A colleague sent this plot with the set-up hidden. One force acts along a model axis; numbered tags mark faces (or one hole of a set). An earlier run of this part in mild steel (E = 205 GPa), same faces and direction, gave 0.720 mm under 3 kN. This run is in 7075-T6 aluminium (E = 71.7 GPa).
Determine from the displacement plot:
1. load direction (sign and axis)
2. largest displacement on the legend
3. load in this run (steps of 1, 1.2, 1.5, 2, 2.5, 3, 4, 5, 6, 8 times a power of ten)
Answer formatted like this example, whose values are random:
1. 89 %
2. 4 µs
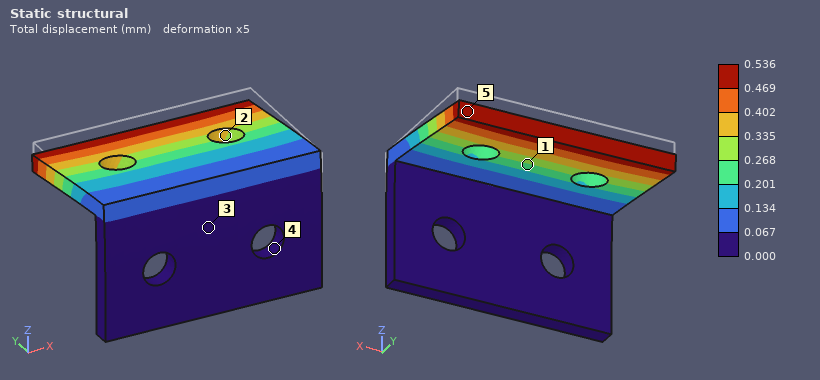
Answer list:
1. -Z
2. 0.536 mm
3. 800 N
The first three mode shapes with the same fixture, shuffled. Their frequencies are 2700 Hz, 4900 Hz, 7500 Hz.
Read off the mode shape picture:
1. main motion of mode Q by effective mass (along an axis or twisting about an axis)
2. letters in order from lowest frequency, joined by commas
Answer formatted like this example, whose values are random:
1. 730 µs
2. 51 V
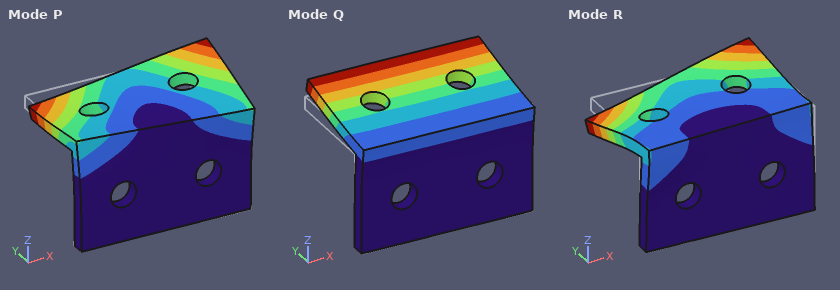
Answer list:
1. along Z
2. Q, P, R
